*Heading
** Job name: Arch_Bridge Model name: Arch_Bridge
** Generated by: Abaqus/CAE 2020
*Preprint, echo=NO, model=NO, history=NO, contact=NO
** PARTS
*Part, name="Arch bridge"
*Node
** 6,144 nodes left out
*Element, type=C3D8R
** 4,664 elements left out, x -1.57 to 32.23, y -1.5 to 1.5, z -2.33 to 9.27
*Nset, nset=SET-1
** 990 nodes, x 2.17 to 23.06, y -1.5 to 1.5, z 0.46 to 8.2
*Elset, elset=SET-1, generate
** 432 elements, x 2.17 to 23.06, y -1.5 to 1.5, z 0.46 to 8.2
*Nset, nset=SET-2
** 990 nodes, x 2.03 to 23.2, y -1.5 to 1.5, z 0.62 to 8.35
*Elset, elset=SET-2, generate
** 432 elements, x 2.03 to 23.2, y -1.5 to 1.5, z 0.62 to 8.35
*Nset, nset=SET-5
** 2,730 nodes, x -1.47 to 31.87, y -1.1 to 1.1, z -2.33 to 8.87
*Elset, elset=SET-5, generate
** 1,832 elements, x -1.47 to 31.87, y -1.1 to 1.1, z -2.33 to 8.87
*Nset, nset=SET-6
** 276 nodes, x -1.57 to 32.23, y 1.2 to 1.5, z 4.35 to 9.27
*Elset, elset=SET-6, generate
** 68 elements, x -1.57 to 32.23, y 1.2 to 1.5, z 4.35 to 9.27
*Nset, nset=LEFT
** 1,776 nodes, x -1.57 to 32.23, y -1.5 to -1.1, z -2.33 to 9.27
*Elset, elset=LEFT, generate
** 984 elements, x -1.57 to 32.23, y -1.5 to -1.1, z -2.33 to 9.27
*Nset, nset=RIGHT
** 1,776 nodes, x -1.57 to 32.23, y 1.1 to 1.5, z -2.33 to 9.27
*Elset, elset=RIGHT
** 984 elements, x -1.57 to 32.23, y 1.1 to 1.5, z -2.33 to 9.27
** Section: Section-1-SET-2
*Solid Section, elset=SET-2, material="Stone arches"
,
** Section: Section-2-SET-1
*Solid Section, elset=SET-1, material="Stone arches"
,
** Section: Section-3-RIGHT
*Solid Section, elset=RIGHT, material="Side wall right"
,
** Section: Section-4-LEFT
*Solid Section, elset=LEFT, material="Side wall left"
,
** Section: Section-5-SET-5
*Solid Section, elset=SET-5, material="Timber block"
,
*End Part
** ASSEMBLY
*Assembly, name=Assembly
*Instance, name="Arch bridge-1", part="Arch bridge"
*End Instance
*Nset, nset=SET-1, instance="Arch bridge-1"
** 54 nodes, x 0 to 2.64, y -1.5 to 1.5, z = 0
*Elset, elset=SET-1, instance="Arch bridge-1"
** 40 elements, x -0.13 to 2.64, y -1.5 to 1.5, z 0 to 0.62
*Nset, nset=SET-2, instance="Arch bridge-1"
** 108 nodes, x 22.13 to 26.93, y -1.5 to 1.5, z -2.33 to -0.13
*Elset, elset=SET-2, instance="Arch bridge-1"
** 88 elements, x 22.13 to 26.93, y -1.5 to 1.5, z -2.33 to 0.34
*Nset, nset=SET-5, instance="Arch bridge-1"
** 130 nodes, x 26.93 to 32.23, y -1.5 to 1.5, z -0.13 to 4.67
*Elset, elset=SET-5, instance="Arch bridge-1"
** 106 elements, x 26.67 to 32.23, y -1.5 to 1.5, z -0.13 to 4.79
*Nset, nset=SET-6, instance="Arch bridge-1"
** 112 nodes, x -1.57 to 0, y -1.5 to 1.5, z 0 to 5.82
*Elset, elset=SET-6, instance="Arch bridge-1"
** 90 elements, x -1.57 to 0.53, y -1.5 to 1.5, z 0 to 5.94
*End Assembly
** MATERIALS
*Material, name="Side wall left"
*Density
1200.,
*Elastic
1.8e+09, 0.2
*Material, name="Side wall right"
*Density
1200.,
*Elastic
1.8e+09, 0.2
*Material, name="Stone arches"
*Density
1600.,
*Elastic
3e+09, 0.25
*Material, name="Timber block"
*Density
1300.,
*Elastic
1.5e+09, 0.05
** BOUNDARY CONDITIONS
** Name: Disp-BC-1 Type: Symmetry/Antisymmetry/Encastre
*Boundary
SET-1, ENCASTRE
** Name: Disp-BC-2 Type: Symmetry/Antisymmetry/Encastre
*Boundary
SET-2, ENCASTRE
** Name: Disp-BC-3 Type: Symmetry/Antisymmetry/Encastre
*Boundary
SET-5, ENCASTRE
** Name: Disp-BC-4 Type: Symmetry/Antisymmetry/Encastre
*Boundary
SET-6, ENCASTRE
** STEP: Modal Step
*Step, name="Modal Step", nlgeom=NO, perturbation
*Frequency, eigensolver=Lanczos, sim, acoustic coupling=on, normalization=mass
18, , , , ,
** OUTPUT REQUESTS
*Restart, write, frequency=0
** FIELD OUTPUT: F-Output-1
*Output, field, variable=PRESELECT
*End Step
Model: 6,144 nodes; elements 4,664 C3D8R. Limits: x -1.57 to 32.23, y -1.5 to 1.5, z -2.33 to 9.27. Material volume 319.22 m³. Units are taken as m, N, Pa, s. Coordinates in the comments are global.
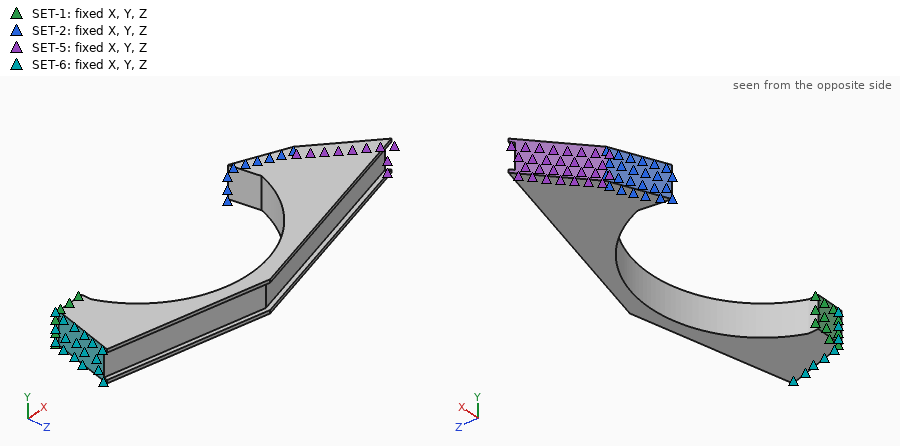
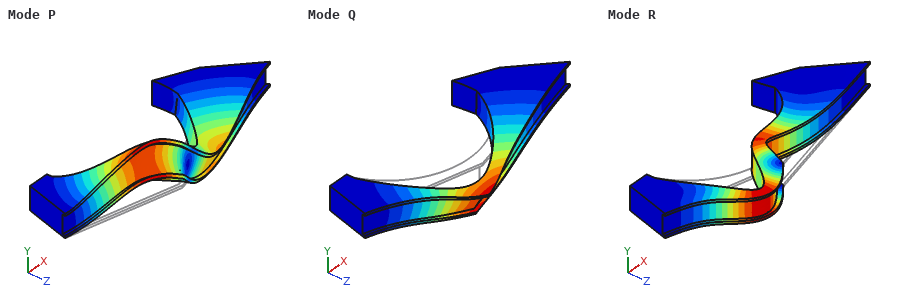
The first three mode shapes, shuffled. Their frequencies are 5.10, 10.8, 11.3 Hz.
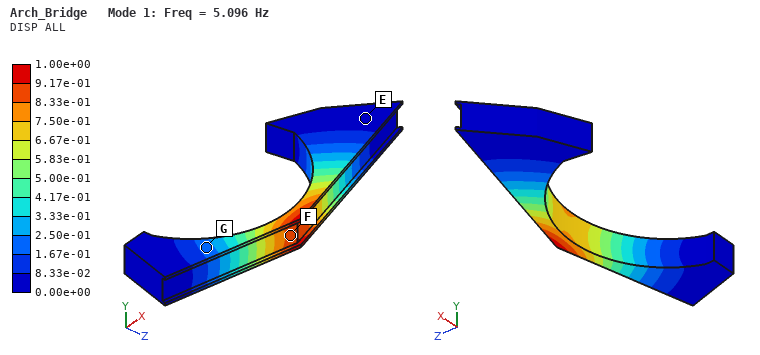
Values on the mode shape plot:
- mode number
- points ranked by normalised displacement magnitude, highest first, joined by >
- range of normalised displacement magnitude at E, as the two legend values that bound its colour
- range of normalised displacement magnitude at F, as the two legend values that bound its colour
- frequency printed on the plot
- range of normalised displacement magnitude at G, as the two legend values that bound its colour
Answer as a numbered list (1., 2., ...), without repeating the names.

1. 1
2. F > G > E
3. 0.00e+00 to 8.33e-02
4. 8.33e-01 to 9.17e-01
5. 5.096 Hz
6. 1.67e-01 to 2.50e-01
